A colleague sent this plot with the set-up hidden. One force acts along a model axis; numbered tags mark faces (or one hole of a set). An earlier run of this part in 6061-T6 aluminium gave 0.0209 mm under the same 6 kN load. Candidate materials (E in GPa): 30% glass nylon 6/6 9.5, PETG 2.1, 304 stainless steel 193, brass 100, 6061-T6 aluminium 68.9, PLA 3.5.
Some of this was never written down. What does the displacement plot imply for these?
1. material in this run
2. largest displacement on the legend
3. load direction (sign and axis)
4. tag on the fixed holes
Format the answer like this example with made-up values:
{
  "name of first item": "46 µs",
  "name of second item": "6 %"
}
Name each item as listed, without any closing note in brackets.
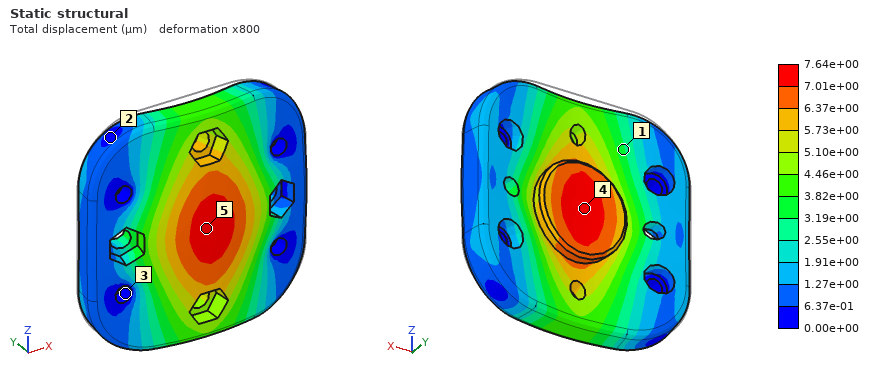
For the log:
{
  "material in this run": "304 stainless steel",
  "largest displacement on the legend": "7.64e+00 µm",
  "load direction": "-Y",
  "tag on the fixed holes": "3"
}
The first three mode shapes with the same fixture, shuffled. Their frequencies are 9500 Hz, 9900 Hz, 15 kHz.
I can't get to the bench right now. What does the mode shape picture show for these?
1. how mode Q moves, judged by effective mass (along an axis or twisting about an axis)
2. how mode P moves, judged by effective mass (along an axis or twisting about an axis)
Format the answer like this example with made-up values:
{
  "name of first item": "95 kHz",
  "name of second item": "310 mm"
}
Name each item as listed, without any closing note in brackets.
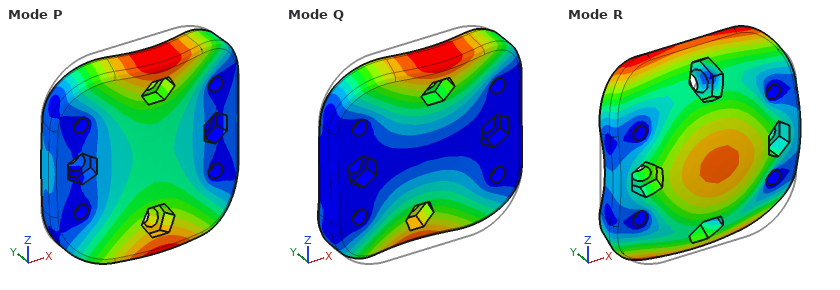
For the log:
{
  "how mode Q moves, judged by effective mass": "twisting about X",
  "how mode P moves, judged by effective mass": "along Y"
}
